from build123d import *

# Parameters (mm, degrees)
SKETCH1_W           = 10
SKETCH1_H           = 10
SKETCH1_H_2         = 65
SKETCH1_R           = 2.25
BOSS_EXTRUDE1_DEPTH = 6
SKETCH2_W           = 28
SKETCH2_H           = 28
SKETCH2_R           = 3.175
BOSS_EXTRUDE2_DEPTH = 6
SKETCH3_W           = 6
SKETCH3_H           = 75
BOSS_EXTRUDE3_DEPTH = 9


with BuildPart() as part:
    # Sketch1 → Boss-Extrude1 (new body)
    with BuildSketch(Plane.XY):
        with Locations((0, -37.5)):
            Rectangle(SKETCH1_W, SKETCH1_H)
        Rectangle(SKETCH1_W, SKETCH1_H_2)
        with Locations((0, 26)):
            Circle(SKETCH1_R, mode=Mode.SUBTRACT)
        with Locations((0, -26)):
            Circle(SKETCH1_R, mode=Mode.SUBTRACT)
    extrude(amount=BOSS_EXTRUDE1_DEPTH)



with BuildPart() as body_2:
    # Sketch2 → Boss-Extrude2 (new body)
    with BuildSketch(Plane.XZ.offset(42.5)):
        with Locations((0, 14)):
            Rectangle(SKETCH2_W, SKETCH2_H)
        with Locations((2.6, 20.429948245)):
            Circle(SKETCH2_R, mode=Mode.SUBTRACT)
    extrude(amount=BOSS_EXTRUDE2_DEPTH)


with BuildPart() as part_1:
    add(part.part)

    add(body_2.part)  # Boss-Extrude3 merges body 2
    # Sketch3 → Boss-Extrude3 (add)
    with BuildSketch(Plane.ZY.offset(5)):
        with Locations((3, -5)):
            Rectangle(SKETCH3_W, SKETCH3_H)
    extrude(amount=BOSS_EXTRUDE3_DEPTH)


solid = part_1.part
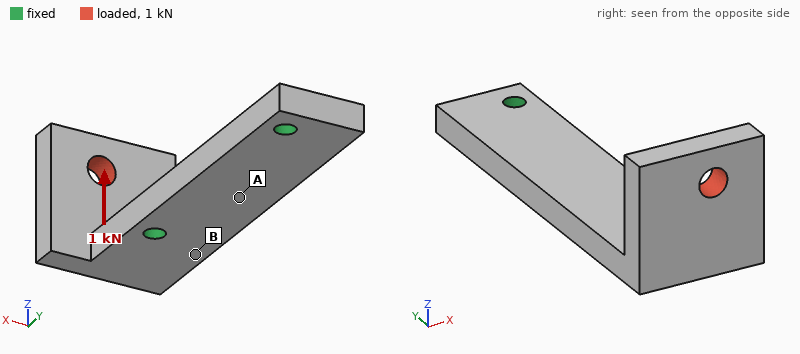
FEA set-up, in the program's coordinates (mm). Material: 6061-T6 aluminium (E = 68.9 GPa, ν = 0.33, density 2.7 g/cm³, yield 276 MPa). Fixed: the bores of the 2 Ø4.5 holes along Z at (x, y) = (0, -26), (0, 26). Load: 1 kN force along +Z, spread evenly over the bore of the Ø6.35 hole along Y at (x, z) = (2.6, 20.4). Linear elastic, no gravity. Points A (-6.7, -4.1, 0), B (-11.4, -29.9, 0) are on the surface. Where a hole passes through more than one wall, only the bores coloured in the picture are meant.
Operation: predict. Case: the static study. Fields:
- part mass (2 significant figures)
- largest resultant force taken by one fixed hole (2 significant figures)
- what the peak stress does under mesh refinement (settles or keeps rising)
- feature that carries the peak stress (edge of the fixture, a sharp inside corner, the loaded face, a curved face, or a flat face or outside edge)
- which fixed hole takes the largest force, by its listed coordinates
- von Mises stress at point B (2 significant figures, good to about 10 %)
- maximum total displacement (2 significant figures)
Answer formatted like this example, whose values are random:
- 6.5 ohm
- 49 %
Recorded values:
- 35 g
- 1.0 kN
- keeps rising
- edge of the fixture
- (0, -26)
- 76 MPa
- 0.29 mm
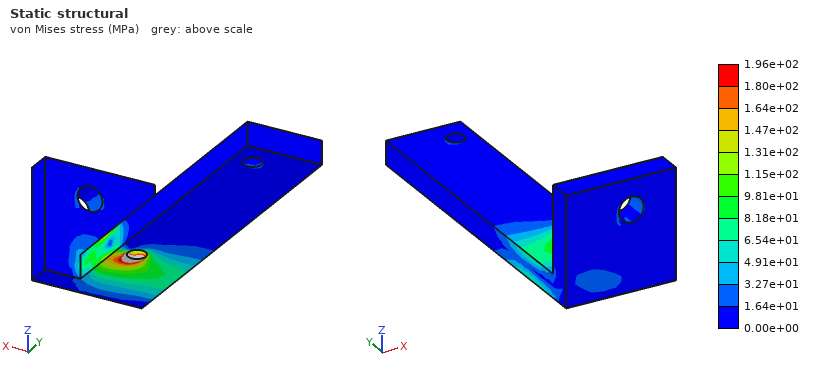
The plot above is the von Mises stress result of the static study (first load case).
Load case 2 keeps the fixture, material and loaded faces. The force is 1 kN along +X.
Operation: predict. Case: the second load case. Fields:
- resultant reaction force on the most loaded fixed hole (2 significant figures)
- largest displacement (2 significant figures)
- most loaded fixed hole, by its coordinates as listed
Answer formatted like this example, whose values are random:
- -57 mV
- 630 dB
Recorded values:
- 1.3 kN
- 0.34 mm
- (0, -26)
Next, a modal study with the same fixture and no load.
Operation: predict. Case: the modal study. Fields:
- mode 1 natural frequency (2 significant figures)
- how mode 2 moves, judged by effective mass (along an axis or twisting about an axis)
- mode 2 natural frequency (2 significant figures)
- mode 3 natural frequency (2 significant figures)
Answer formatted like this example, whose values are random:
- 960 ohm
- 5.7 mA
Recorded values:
- 2800 Hz
- along X
- 3500 Hz
- 7900 Hz
